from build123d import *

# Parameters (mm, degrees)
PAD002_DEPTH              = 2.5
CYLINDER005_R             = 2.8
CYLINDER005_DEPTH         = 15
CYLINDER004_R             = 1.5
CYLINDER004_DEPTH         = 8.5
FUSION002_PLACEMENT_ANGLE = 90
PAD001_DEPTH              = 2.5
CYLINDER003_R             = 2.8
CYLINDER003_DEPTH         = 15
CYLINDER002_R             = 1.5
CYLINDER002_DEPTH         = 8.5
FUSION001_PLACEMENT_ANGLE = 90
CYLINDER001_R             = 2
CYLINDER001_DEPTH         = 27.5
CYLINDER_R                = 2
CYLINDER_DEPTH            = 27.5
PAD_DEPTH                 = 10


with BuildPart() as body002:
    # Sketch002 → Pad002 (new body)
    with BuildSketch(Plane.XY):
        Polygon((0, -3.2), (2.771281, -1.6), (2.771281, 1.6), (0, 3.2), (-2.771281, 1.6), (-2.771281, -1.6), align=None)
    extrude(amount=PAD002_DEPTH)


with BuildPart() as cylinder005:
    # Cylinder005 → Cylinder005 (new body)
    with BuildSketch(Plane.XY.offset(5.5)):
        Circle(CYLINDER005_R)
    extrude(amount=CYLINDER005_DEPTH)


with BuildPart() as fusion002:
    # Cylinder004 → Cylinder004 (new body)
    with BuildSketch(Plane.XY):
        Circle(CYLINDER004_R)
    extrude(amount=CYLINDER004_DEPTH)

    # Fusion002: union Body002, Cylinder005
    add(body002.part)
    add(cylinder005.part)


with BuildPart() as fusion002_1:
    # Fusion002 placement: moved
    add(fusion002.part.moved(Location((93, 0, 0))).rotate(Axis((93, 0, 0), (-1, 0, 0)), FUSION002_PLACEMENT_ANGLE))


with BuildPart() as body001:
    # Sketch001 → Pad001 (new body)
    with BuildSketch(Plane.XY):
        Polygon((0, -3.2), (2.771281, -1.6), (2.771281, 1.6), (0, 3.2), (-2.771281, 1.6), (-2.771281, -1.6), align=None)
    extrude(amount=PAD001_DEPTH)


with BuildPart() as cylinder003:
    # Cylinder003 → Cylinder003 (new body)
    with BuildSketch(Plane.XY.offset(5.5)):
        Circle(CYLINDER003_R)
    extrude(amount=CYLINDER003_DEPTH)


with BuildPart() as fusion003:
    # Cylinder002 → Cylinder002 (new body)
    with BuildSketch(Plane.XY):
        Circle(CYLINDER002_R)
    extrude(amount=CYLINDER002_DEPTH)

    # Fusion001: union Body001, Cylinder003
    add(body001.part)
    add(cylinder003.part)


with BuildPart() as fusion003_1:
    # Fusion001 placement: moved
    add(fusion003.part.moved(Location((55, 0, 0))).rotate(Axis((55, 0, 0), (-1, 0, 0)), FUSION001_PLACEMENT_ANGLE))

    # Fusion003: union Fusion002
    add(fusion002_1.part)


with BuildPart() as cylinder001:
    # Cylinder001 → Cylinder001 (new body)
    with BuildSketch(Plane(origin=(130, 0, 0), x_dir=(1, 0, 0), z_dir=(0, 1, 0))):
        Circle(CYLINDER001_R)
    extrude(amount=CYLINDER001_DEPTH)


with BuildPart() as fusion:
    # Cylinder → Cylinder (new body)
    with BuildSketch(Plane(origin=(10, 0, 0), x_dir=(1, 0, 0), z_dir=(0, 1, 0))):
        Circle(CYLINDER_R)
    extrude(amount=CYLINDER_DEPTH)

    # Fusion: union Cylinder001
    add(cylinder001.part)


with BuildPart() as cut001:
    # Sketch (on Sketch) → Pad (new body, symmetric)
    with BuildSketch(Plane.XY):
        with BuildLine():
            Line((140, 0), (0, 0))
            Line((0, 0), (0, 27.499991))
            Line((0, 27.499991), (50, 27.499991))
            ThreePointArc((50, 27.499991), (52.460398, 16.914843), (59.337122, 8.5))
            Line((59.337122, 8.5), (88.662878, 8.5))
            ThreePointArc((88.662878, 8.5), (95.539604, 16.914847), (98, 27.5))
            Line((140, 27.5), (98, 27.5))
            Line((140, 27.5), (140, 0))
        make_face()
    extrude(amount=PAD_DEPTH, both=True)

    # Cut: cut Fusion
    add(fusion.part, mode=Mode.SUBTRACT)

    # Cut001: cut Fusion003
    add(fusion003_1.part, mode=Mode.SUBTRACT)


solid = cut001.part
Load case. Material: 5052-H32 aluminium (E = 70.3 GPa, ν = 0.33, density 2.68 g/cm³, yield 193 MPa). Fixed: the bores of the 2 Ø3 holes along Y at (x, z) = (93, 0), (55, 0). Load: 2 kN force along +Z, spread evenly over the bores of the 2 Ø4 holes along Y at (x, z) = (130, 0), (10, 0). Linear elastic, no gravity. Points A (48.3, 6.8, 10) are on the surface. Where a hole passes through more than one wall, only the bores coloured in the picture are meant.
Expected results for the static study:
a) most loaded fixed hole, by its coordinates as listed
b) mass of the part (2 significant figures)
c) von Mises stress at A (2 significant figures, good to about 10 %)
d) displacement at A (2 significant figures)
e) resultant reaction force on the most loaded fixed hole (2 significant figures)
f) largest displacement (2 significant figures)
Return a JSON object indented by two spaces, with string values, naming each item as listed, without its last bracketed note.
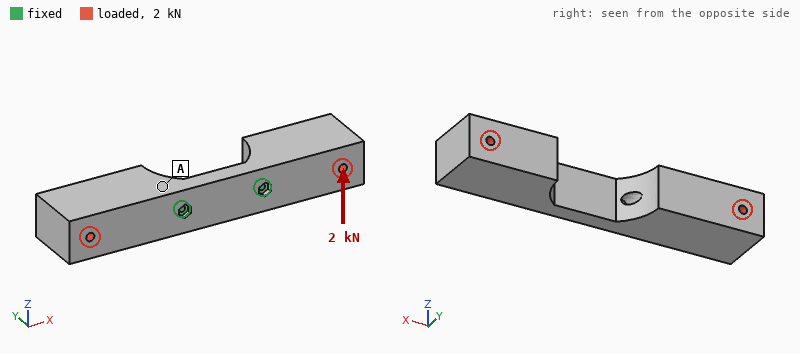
{
  "most loaded fixed hole, by its coordinates as listed": "(55, 0)",
  "mass of the part": "160 g",
  "von Mises stress at A": "41 MPa",
  "displacement at A": "0.062 mm",
  "resultant reaction force on the most loaded fixed hole": "1.2 kN",
  "largest displacement": "0.28 mm"
}
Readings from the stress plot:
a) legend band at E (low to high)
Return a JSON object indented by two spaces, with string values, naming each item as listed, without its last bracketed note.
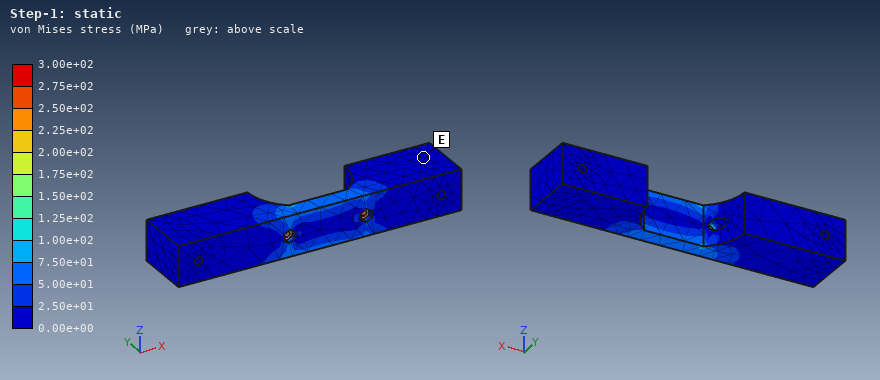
{
  "legend band at E": "0.00e+00 to 2.50e+01 MPa"
}
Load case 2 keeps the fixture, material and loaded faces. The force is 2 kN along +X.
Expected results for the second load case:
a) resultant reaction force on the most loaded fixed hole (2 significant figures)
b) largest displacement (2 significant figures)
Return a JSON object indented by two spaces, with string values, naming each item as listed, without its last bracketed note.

{
  "resultant reaction force on the most loaded fixed hole": "1.1 kN",
  "largest displacement": "70 µm"
}
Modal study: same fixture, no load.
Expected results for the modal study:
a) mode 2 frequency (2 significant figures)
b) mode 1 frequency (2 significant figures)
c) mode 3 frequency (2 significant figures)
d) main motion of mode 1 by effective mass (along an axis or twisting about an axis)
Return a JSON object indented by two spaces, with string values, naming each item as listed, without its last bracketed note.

{
  "mode 2 frequency": "1600 Hz",
  "mode 1 frequency": "1200 Hz",
  "mode 3 frequency": "1700 Hz",
  "main motion of mode 1 by effective mass": "along Y"
}
